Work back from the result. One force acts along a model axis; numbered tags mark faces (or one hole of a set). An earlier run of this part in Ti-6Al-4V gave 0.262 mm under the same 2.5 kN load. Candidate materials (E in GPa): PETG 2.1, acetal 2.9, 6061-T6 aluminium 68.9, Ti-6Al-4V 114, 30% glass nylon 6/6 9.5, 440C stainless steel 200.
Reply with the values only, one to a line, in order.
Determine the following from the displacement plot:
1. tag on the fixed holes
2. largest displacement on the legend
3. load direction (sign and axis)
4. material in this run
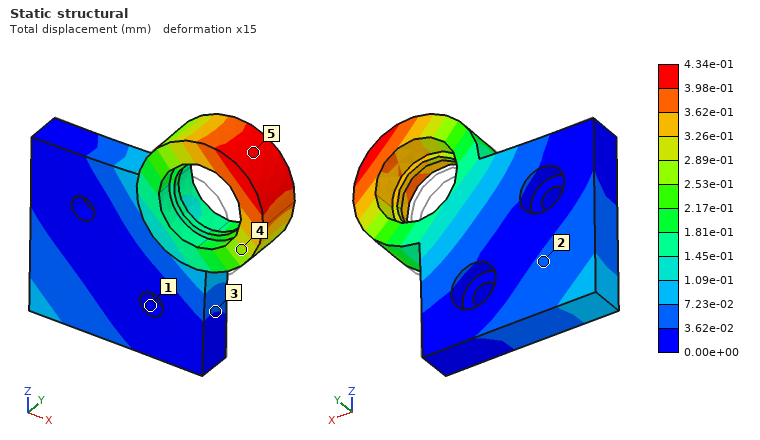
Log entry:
1
4.34e-01 mm
+Y
6061-T6 aluminium
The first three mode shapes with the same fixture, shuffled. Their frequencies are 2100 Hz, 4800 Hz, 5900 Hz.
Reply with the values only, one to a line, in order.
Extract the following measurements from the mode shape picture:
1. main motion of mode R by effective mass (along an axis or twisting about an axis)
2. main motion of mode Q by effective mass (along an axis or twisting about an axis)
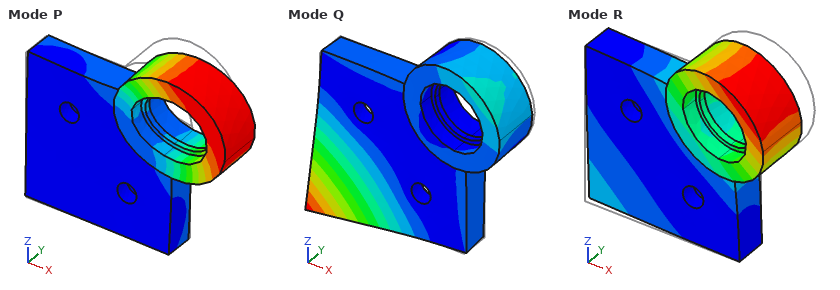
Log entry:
along Y
along Y
